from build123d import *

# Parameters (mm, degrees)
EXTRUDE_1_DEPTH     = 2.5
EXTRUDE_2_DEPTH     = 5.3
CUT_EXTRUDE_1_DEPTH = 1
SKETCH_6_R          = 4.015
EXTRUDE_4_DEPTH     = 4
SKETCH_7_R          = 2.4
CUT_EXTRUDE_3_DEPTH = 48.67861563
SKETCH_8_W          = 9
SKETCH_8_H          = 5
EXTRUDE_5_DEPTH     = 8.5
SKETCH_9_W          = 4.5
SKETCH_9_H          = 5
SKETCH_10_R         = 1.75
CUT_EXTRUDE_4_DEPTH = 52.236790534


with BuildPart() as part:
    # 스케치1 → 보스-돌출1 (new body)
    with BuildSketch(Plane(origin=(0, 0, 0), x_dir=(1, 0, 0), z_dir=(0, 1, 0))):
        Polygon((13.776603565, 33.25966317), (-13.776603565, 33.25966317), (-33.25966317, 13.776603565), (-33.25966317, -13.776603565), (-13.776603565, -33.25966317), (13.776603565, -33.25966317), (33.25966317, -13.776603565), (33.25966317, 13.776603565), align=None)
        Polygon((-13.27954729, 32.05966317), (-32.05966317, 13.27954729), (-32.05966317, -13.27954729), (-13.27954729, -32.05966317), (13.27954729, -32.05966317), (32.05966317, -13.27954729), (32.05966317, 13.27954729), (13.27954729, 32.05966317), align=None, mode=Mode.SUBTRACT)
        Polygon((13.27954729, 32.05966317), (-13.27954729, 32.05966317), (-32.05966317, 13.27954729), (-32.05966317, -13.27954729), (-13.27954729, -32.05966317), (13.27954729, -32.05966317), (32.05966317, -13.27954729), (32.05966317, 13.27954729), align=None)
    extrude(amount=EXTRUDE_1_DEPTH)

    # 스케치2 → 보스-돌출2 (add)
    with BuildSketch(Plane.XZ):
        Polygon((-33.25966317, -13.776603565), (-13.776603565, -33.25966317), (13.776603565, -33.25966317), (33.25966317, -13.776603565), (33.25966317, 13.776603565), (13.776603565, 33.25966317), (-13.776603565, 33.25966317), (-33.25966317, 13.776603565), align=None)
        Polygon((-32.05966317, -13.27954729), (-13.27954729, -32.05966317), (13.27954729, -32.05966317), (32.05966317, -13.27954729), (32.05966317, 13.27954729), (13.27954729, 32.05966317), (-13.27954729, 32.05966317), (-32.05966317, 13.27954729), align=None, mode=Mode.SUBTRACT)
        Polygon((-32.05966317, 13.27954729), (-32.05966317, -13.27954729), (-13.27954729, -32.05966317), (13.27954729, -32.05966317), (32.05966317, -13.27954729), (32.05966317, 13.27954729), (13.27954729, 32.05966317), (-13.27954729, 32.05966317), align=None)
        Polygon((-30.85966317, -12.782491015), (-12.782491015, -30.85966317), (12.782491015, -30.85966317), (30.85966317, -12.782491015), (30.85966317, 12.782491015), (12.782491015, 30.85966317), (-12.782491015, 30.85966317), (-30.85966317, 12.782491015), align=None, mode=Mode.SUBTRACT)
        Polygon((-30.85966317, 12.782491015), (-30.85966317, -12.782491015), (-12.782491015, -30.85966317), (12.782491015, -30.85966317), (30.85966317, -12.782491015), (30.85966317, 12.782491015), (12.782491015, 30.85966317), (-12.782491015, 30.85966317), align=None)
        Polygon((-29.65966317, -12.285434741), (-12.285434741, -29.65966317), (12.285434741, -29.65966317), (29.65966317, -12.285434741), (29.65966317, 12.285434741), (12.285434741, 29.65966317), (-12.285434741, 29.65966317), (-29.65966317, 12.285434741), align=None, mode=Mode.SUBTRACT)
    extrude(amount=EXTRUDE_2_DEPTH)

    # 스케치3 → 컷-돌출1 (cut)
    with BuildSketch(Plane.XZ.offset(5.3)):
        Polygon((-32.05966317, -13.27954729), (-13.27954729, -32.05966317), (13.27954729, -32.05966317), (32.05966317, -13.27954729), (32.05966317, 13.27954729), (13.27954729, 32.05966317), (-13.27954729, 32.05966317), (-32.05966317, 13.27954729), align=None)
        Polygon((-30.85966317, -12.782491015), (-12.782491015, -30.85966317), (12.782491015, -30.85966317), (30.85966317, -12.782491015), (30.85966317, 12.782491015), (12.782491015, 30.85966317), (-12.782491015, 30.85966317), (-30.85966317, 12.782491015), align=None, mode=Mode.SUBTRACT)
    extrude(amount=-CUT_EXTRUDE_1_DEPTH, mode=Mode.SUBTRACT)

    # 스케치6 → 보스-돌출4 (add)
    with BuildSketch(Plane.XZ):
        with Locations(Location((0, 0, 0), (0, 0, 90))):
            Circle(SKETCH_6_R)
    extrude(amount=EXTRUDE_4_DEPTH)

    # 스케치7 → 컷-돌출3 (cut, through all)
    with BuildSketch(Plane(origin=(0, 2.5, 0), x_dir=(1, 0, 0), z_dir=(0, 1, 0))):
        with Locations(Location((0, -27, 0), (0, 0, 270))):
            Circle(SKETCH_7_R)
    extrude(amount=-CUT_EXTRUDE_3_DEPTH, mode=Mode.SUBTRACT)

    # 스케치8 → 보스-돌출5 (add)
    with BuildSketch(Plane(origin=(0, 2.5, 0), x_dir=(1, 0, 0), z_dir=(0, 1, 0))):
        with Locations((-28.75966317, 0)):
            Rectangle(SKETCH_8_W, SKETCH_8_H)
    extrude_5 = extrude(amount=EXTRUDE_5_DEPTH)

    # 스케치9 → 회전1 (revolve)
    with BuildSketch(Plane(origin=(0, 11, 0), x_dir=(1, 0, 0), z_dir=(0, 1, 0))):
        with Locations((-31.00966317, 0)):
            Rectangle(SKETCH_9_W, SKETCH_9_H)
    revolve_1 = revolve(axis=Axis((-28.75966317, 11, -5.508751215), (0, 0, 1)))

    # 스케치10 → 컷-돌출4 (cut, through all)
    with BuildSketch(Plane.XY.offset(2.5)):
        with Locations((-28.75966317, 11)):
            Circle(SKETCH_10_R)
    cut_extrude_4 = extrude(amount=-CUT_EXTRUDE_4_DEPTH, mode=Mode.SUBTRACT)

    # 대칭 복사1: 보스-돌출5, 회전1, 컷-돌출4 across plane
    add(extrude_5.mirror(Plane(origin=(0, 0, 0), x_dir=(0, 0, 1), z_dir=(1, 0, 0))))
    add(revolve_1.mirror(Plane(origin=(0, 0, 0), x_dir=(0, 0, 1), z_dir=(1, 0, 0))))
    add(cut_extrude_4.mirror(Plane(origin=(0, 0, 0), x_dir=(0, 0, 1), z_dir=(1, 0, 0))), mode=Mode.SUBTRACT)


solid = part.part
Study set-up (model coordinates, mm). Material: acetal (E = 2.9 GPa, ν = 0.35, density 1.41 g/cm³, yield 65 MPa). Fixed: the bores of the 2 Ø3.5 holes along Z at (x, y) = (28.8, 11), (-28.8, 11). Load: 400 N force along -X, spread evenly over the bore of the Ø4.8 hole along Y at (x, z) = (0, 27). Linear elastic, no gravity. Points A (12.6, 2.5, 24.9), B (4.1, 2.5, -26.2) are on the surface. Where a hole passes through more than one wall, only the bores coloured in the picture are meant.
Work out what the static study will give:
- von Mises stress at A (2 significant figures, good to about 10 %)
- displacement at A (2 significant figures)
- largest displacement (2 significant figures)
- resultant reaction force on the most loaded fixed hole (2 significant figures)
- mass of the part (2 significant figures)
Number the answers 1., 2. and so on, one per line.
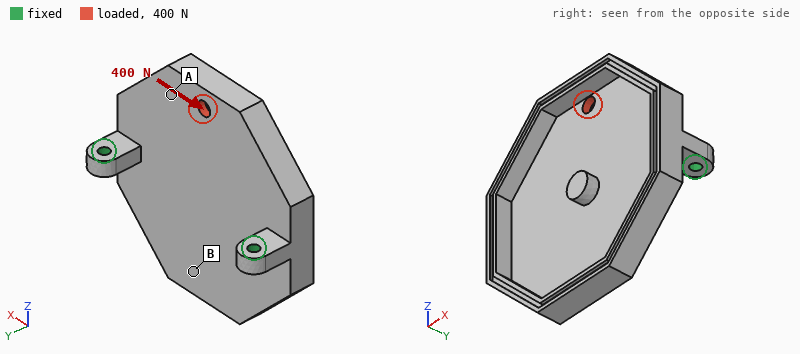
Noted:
1. 6.9 MPa
2. 0.38 mm
3. 0.46 mm
4. 270 N
5. 20 g
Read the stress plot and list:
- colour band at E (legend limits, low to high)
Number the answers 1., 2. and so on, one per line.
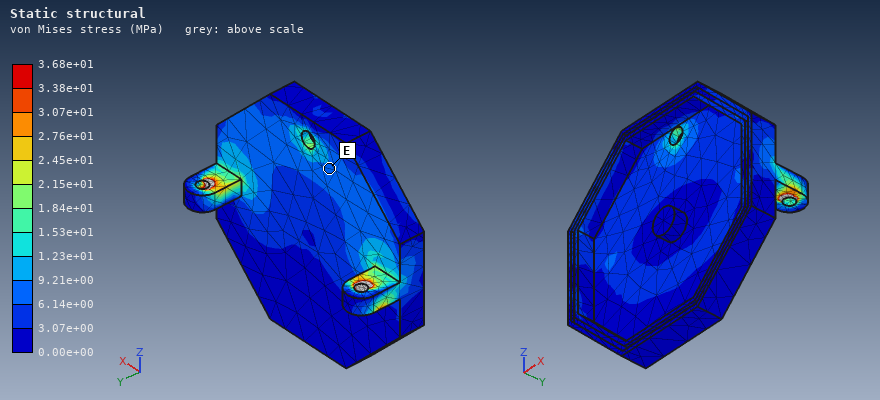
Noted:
1. 6.14e+00 to 9.21e+00 MPa
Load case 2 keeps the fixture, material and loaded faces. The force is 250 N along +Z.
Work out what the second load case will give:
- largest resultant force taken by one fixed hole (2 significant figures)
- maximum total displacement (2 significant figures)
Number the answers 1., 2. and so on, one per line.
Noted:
1. 130 N
2. 0.70 mm
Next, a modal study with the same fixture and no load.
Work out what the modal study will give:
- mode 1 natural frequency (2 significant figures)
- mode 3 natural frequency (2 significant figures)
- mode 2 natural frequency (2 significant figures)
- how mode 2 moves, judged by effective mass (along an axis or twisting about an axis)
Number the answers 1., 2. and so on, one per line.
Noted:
1. 390 Hz
2. 1200 Hz
3. 780 Hz
4. along Y
